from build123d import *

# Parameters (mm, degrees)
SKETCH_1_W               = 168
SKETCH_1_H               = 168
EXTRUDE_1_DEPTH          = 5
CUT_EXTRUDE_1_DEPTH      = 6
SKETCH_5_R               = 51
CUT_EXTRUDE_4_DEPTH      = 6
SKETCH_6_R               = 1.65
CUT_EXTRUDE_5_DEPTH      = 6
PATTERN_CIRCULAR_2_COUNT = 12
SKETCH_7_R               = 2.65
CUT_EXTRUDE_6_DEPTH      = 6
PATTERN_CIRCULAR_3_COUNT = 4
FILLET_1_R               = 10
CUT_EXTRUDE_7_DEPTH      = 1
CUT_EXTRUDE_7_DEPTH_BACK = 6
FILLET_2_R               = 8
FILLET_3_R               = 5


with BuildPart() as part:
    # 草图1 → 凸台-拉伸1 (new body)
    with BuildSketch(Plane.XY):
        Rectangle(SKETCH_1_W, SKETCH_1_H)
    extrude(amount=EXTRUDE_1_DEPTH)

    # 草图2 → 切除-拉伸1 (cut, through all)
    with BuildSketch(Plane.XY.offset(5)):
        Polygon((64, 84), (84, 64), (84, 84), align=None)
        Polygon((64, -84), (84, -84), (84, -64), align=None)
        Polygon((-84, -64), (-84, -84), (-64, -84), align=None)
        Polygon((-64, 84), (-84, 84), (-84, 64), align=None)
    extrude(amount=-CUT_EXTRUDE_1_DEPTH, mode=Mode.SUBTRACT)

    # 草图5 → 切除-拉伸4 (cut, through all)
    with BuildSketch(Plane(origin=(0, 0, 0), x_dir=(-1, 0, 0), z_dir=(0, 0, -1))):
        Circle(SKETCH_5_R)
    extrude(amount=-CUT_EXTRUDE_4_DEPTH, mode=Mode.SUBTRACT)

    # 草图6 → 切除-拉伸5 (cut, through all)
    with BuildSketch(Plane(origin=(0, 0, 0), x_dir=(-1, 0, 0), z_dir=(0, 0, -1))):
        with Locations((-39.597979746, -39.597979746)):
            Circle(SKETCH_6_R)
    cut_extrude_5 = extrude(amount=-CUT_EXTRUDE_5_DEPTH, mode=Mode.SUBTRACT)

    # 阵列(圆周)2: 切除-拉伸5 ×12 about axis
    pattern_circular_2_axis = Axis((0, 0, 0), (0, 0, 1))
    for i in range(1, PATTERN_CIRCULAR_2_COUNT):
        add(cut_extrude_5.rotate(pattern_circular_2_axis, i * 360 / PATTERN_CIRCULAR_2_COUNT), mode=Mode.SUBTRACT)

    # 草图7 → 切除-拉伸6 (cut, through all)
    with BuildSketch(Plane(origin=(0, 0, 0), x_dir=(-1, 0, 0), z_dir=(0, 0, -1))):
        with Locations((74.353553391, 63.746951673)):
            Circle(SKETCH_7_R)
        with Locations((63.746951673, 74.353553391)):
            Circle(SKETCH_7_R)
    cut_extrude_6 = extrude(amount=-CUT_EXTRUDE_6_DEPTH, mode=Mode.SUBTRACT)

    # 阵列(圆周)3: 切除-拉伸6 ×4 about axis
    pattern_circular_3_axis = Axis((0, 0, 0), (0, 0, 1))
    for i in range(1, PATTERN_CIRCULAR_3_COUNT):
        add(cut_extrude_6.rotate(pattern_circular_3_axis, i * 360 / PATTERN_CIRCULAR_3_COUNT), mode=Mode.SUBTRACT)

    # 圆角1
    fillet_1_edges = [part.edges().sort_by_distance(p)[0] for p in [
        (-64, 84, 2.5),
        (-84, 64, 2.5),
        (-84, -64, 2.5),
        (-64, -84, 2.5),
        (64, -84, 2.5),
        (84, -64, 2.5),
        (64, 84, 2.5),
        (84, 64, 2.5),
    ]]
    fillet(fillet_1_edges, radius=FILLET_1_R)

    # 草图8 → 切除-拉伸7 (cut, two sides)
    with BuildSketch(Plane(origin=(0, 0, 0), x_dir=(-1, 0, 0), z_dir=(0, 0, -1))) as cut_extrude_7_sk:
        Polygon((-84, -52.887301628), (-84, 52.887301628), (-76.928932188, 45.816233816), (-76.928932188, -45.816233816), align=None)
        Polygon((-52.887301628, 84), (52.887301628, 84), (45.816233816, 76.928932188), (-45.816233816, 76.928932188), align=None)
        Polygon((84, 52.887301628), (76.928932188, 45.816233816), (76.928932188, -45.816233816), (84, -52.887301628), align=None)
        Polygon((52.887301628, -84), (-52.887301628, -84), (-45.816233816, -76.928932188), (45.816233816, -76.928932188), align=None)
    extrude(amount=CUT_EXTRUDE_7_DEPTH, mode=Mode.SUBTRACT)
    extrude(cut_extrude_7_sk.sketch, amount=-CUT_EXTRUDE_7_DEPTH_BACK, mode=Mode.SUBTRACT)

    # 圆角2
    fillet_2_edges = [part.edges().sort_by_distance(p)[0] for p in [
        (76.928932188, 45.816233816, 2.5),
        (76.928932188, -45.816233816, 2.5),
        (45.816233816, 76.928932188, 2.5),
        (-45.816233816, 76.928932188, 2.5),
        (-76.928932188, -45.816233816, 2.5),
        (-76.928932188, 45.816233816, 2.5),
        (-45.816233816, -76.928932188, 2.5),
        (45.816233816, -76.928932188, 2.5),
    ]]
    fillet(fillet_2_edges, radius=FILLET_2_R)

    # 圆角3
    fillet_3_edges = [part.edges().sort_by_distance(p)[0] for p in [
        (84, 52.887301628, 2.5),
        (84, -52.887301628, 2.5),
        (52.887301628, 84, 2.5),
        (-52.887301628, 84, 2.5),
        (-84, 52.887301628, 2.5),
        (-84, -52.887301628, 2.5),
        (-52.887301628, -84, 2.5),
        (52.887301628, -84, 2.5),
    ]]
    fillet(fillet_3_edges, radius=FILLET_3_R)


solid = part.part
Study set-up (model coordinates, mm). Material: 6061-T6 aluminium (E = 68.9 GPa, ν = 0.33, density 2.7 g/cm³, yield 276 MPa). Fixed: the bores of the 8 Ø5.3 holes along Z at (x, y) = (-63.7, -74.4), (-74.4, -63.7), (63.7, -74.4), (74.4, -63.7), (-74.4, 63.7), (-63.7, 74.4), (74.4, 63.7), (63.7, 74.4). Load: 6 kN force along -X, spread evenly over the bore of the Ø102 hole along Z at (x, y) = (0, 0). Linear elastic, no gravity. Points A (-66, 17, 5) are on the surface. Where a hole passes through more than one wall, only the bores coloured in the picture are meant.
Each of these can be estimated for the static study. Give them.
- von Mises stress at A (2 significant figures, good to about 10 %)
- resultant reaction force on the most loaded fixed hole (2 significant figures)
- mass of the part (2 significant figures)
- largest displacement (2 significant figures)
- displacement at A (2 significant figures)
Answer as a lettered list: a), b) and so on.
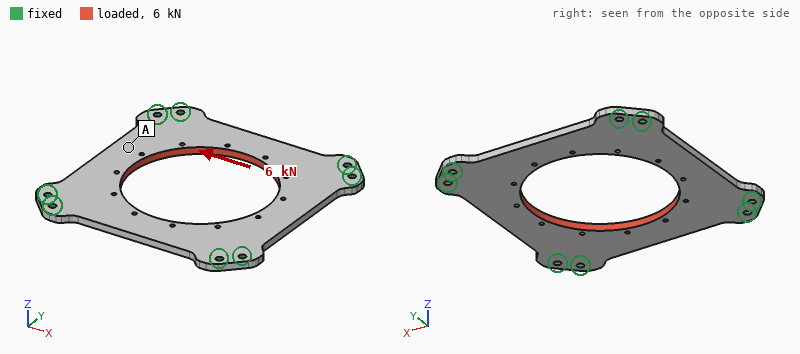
a) 6.1 MPa
b) 1.3 kN
c) 220 g
d) 21 µm
e) 18 µm
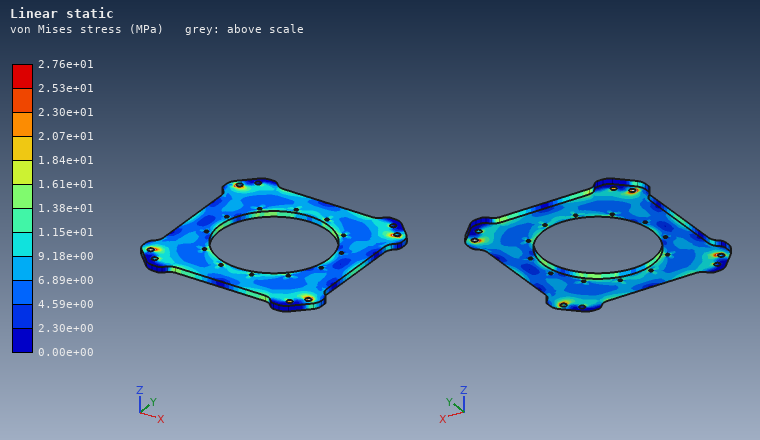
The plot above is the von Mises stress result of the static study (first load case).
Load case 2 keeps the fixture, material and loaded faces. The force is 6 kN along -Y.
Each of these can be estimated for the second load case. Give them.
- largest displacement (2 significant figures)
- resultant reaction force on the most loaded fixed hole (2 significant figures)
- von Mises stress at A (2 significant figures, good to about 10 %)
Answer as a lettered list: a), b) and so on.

a) 21 µm
b) 1.3 kN
c) 7.6 MPa
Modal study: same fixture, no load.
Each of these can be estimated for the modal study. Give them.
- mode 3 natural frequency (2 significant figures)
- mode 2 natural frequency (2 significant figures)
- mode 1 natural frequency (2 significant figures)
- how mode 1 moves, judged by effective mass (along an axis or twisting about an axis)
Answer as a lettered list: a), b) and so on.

a) 1600 Hz
b) 1600 Hz
c) 1400 Hz
d) along Z
